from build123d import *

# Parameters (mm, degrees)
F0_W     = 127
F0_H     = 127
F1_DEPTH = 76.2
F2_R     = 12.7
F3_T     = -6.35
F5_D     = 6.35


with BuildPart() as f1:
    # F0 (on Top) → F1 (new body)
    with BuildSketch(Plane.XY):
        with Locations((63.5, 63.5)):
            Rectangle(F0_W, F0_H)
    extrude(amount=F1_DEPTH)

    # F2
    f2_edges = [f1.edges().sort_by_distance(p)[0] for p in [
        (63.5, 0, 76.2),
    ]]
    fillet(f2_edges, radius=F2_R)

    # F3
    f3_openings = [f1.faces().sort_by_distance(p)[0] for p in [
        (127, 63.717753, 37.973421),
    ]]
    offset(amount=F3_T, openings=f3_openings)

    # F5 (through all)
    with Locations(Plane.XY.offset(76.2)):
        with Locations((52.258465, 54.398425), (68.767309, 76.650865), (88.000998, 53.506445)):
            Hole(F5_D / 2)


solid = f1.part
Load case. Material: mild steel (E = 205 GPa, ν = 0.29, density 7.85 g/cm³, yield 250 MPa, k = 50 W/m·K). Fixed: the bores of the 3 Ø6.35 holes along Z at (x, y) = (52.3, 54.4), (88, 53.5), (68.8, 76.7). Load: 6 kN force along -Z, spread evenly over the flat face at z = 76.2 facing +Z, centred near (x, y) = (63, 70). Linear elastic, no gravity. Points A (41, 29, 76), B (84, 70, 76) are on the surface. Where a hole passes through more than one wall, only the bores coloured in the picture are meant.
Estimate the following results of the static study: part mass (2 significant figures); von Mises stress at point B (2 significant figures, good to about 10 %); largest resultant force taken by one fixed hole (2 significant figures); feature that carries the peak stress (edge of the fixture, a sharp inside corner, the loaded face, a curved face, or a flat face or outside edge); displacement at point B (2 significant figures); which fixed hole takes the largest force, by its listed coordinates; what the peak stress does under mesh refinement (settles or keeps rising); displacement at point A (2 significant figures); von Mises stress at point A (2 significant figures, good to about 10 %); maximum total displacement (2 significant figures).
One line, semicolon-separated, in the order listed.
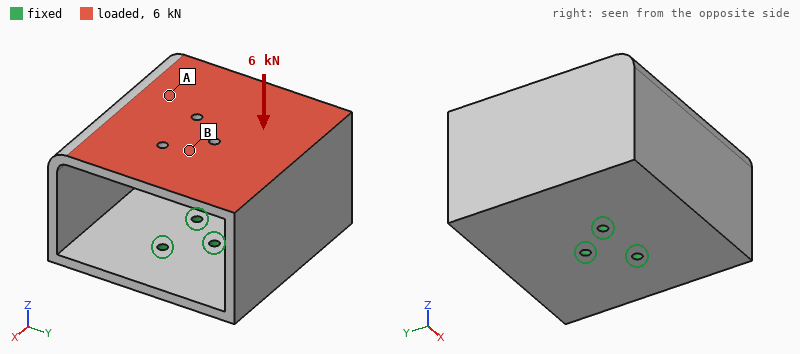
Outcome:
2.7 kg; 43 MPa; 3.2 kN; edge of the fixture; 0.22 mm; (68.8, 76.7); keeps rising; 0.12 mm; 26 MPa; 0.27 mm
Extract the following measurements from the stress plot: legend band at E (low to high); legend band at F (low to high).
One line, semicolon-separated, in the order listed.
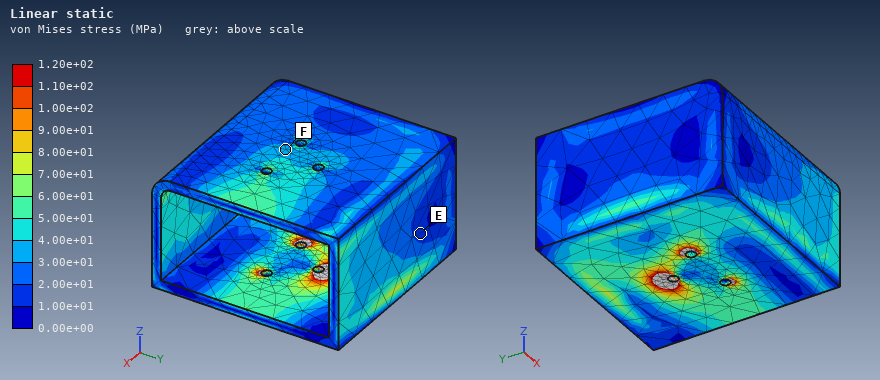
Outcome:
1.00e+01 to 2.00e+01 MPa; 3.00e+01 to 4.00e+01 MPa
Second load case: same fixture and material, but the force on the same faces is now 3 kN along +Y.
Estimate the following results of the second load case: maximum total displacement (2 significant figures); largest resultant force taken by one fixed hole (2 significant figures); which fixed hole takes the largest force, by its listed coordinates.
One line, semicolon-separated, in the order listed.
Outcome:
0.50 mm; 4.6 kN; (68.8, 76.7)
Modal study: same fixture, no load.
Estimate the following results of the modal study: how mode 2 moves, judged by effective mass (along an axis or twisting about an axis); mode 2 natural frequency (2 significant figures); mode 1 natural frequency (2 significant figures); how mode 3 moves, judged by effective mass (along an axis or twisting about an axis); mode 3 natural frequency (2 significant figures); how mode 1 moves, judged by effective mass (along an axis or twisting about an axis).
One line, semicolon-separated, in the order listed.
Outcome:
along X; 420 Hz; 350 Hz; along Z; 790 Hz; along Y
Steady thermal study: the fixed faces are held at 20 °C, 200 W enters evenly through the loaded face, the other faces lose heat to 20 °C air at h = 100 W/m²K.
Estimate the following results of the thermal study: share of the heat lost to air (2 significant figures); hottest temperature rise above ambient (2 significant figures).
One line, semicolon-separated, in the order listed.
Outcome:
97 %; 72 K
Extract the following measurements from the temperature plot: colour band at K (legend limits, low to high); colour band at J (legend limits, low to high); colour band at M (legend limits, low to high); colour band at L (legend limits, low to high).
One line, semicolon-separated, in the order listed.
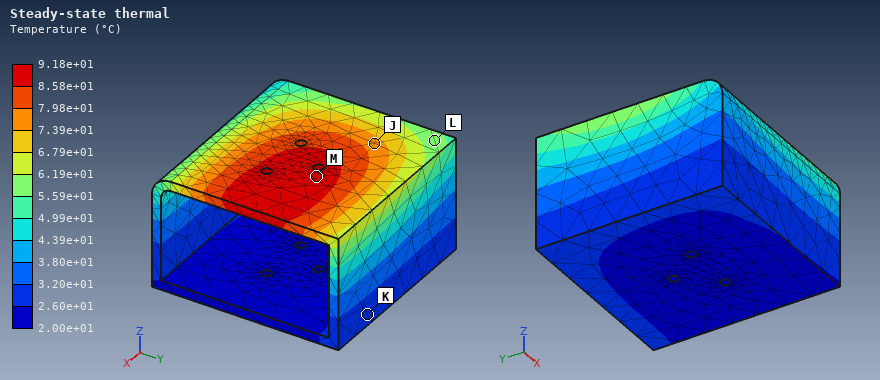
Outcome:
2.60e+01 to 3.20e+01 °C; 7.39e+01 to 7.98e+01 °C; 8.58e+01 to 9.18e+01 °C; 5.59e+01 to 6.19e+01 °C
